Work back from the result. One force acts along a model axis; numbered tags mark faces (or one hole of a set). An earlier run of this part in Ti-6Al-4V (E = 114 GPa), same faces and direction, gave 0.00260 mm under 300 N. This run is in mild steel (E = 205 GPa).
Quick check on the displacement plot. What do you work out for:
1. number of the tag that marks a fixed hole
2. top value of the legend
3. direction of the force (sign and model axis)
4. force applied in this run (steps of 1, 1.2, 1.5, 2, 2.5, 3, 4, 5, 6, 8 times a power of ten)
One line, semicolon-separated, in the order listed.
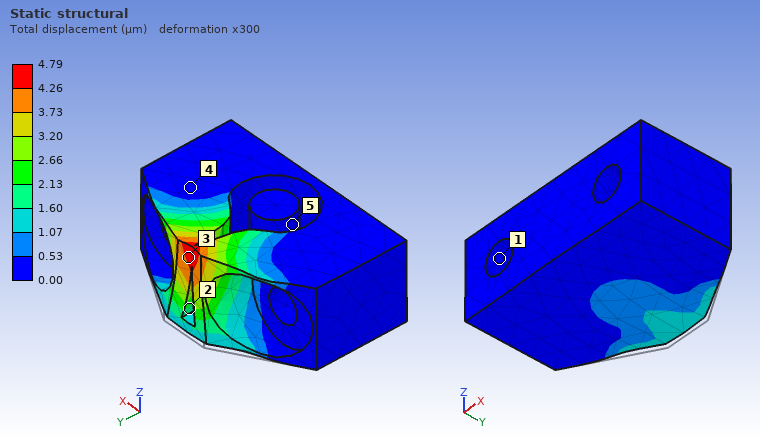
1; 4.79 µm; -Y; 1 kN
